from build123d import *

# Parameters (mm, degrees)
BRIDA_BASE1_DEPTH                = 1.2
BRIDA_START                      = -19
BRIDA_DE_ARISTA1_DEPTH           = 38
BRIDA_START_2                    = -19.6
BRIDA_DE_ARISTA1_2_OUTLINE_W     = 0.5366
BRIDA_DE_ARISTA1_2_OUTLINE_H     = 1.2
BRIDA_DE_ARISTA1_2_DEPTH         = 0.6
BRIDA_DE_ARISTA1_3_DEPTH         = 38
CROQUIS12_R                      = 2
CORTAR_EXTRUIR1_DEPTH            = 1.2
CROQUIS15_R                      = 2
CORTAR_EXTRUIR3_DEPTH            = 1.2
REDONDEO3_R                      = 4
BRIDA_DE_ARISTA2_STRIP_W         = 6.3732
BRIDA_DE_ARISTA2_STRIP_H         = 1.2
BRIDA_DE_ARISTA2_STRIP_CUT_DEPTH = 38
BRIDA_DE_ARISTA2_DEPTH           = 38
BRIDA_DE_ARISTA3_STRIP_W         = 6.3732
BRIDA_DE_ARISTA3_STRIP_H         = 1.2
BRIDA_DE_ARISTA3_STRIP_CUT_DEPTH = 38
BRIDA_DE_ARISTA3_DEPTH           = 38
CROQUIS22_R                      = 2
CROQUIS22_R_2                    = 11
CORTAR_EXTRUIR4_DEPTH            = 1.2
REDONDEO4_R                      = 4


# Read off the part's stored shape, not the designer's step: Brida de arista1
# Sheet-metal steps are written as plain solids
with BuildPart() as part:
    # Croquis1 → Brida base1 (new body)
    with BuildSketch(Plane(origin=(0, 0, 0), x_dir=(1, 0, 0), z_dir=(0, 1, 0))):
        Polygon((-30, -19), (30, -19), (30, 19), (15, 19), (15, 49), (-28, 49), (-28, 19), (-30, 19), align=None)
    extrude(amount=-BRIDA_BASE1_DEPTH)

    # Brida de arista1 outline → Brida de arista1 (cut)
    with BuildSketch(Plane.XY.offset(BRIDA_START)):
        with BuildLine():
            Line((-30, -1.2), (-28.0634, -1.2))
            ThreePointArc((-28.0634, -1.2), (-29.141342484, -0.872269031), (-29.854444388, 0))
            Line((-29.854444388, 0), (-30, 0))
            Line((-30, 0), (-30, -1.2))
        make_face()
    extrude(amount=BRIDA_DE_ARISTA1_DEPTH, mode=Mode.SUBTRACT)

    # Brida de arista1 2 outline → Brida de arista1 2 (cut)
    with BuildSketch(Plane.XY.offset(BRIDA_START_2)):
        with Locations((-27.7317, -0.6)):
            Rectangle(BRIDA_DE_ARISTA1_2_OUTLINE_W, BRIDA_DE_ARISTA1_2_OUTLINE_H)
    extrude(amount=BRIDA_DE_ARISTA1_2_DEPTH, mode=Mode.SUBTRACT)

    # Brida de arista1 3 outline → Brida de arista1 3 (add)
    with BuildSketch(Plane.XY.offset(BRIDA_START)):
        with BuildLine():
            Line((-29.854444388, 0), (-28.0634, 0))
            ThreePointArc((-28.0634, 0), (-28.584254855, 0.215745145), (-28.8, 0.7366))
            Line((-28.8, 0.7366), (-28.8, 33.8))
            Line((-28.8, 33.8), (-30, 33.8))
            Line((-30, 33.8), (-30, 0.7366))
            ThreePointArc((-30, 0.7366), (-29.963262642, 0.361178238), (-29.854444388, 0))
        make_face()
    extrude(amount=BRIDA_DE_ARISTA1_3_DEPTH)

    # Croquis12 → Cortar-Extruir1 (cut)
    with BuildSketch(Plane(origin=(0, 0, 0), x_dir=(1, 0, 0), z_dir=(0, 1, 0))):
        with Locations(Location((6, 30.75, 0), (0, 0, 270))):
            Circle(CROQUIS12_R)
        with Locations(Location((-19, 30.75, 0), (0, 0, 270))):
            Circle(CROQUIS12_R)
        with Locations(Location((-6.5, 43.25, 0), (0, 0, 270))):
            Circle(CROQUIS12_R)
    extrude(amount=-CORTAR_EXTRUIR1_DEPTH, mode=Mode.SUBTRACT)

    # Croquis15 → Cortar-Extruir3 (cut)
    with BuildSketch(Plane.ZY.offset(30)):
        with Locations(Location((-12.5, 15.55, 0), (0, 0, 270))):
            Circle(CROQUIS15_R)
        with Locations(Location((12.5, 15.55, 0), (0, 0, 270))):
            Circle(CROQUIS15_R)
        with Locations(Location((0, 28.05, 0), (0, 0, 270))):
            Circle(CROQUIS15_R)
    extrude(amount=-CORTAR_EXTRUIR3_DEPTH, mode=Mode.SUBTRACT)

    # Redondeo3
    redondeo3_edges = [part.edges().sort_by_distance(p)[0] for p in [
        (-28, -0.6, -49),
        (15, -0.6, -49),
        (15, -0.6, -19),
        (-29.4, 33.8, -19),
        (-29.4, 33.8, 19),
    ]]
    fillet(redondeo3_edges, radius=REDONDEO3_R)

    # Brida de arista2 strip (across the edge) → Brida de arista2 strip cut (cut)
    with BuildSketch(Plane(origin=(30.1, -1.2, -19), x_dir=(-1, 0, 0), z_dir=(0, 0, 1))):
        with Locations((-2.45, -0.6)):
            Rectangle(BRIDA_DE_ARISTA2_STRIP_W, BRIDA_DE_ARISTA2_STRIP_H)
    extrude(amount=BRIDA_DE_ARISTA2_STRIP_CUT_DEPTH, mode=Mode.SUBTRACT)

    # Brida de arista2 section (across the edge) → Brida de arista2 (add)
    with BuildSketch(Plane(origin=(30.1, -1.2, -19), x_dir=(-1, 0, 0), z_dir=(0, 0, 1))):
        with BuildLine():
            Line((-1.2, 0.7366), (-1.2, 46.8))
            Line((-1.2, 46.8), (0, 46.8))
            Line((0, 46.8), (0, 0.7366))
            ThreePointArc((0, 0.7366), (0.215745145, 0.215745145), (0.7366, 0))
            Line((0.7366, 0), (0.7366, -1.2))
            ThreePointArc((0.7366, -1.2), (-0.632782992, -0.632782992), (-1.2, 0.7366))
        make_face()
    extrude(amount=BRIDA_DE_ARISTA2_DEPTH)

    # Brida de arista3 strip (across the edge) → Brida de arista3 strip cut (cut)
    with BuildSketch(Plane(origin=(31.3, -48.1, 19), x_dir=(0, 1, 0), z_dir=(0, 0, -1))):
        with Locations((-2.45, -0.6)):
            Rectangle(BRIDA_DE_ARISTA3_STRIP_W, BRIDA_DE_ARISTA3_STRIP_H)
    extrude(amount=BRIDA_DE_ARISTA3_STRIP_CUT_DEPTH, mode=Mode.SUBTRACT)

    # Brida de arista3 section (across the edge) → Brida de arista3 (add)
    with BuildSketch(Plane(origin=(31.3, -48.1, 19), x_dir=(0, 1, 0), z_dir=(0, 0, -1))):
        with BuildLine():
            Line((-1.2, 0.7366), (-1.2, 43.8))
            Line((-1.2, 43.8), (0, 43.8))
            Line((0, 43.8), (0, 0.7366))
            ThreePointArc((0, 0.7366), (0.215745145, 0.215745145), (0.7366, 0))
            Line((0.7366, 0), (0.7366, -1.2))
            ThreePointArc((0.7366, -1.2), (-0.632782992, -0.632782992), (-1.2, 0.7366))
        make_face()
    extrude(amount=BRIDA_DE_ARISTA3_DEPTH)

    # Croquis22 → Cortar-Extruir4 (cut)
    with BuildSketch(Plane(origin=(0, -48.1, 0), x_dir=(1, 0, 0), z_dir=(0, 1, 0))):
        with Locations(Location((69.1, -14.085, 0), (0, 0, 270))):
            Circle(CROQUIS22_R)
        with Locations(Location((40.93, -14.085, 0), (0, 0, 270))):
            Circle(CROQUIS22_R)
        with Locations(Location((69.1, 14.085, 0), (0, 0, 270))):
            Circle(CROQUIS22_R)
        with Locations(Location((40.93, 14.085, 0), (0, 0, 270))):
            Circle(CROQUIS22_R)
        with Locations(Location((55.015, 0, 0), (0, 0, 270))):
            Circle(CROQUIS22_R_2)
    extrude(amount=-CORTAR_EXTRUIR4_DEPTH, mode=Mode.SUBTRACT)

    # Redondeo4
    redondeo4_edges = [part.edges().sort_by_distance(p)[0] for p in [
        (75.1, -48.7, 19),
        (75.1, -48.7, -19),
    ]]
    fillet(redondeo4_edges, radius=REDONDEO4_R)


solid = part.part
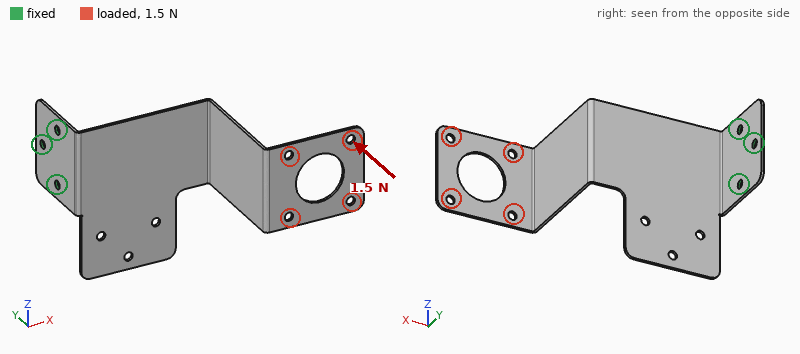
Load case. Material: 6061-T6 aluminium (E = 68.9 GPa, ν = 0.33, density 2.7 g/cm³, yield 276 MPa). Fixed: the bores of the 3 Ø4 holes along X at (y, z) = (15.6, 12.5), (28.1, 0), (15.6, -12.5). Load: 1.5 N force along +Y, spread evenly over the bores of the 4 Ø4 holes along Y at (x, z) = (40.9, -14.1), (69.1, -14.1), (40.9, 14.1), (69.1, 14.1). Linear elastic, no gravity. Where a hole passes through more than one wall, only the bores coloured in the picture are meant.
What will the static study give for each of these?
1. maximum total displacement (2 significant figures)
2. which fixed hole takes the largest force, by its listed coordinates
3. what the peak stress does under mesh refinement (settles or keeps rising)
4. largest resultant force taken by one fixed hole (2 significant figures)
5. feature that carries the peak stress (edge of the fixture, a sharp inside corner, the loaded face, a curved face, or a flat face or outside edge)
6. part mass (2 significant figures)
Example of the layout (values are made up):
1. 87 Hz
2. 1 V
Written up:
1. 1.8 mm
2. (28.1, 0)
3. keeps rising
4. 2.2 N
5. a sharp inside corner
6. 25 g
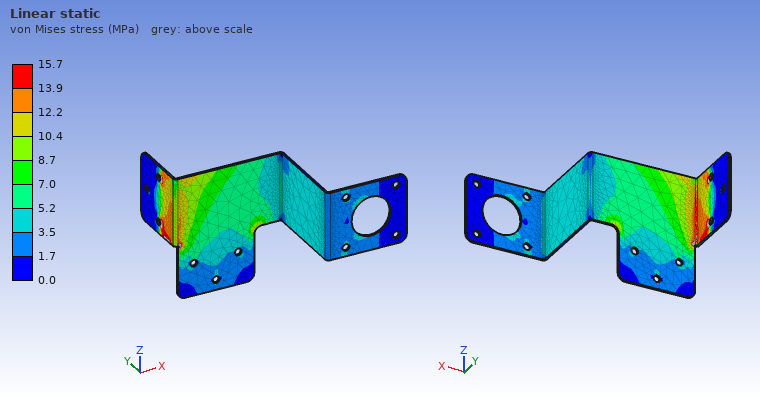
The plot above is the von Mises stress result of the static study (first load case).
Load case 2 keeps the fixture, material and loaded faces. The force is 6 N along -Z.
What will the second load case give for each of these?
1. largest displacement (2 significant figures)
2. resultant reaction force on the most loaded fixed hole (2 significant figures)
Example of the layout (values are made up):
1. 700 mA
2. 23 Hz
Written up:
1. 1.6 mm
2. 24 N
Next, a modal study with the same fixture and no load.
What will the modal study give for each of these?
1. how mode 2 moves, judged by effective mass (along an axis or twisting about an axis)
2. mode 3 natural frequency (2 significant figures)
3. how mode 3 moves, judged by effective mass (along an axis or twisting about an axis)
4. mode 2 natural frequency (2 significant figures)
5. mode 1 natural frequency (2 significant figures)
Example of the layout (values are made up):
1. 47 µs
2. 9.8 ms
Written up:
1. along Z
2. 210 Hz
3. along Y
4. 140 Hz
5. 58 Hz
